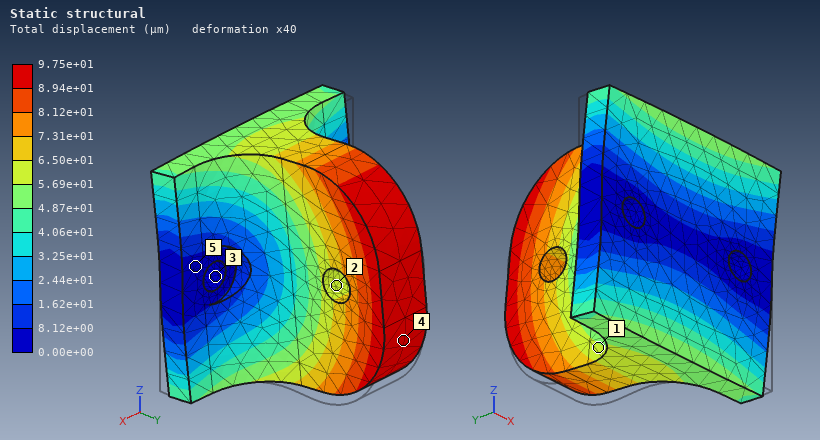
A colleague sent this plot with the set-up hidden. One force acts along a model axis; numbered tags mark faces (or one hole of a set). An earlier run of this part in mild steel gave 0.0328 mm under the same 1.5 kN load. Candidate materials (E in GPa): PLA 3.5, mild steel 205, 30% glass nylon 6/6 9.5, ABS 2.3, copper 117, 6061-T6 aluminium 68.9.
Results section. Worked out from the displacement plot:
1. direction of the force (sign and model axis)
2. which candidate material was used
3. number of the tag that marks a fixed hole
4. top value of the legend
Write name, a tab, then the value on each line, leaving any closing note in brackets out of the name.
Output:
direction of the force	+Z
which candidate material was used	6061-T6 aluminium
number of the tag that marks a fixed hole	3
top value of the legend	9.75e+01 µm
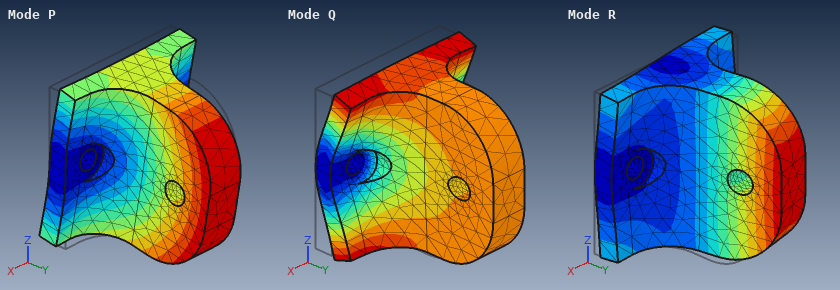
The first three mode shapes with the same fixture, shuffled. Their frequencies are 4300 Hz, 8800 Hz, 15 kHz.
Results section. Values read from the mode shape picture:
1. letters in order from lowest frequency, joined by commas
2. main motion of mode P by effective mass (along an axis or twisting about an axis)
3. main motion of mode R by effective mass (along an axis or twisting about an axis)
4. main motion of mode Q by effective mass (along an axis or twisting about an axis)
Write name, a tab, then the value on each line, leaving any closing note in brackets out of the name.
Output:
letters in order from lowest frequency, joined by commas	P, R, Q
main motion of mode P by effective mass	along Z
main motion of mode R by effective mass	along X
main motion of mode Q by effective mass	along Y
